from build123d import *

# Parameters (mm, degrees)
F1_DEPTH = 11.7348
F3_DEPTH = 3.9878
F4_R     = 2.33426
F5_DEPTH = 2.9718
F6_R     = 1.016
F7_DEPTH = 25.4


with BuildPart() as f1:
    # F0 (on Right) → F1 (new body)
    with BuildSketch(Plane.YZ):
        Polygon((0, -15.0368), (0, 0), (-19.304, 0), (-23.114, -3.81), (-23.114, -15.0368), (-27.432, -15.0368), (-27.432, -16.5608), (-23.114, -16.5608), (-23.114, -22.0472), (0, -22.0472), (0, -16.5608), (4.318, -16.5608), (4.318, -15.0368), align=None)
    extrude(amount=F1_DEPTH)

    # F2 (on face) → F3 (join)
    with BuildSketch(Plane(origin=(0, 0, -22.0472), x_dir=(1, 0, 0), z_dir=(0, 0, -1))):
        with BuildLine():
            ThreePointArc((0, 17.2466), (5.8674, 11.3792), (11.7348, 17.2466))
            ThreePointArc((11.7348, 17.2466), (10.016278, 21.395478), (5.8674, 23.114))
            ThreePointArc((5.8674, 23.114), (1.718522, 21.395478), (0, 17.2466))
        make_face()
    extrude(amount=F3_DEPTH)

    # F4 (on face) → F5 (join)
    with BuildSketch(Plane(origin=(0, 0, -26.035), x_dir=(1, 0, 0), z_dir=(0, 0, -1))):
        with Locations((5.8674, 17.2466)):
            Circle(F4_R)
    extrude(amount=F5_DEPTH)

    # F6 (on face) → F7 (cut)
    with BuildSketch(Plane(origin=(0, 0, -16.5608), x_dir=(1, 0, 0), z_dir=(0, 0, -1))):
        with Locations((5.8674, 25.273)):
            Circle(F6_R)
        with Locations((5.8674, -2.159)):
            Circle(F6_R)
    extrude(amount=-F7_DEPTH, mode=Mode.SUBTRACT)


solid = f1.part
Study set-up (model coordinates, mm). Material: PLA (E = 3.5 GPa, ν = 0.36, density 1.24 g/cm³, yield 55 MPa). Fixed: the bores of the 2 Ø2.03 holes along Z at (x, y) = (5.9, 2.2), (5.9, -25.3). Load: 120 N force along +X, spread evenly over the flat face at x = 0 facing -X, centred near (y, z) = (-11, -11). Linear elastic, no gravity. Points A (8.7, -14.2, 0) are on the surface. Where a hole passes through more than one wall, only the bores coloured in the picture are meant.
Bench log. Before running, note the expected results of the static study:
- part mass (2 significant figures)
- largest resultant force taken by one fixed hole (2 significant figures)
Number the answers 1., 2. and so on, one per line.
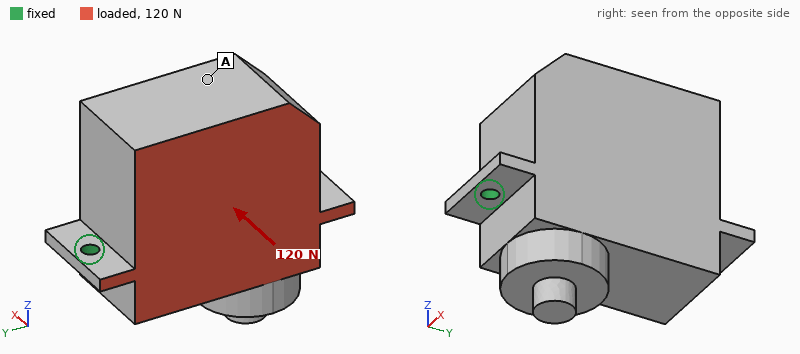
1. 8.1 g
2. 61 N
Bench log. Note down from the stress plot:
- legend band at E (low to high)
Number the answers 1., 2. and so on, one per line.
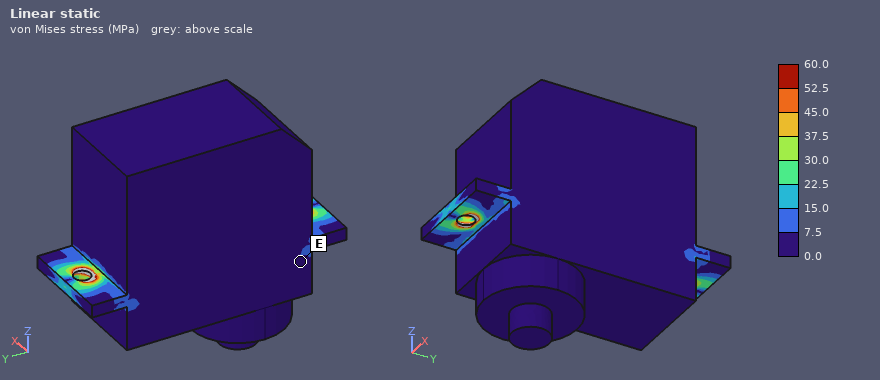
1. 0.0 to 7.5 MPa
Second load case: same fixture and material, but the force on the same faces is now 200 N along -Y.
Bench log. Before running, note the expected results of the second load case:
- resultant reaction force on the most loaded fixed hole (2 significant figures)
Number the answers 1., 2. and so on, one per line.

1. 110 N
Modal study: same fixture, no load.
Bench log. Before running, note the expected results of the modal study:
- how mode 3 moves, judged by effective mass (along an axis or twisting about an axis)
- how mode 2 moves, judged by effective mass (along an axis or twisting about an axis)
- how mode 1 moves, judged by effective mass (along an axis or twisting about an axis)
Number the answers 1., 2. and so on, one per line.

1. along Y
2. along Z
3. along X
